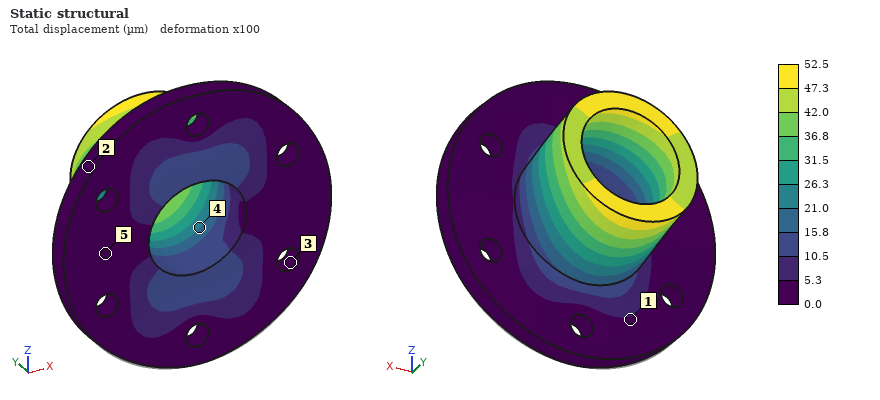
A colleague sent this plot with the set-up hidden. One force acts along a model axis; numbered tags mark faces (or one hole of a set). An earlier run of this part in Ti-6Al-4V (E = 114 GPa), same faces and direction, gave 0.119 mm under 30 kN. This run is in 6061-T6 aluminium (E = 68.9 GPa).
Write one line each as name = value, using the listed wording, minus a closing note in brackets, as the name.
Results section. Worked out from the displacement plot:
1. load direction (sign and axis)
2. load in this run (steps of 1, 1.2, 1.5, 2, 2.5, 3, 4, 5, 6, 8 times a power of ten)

load direction = +Z
load in this run = 8 kN
